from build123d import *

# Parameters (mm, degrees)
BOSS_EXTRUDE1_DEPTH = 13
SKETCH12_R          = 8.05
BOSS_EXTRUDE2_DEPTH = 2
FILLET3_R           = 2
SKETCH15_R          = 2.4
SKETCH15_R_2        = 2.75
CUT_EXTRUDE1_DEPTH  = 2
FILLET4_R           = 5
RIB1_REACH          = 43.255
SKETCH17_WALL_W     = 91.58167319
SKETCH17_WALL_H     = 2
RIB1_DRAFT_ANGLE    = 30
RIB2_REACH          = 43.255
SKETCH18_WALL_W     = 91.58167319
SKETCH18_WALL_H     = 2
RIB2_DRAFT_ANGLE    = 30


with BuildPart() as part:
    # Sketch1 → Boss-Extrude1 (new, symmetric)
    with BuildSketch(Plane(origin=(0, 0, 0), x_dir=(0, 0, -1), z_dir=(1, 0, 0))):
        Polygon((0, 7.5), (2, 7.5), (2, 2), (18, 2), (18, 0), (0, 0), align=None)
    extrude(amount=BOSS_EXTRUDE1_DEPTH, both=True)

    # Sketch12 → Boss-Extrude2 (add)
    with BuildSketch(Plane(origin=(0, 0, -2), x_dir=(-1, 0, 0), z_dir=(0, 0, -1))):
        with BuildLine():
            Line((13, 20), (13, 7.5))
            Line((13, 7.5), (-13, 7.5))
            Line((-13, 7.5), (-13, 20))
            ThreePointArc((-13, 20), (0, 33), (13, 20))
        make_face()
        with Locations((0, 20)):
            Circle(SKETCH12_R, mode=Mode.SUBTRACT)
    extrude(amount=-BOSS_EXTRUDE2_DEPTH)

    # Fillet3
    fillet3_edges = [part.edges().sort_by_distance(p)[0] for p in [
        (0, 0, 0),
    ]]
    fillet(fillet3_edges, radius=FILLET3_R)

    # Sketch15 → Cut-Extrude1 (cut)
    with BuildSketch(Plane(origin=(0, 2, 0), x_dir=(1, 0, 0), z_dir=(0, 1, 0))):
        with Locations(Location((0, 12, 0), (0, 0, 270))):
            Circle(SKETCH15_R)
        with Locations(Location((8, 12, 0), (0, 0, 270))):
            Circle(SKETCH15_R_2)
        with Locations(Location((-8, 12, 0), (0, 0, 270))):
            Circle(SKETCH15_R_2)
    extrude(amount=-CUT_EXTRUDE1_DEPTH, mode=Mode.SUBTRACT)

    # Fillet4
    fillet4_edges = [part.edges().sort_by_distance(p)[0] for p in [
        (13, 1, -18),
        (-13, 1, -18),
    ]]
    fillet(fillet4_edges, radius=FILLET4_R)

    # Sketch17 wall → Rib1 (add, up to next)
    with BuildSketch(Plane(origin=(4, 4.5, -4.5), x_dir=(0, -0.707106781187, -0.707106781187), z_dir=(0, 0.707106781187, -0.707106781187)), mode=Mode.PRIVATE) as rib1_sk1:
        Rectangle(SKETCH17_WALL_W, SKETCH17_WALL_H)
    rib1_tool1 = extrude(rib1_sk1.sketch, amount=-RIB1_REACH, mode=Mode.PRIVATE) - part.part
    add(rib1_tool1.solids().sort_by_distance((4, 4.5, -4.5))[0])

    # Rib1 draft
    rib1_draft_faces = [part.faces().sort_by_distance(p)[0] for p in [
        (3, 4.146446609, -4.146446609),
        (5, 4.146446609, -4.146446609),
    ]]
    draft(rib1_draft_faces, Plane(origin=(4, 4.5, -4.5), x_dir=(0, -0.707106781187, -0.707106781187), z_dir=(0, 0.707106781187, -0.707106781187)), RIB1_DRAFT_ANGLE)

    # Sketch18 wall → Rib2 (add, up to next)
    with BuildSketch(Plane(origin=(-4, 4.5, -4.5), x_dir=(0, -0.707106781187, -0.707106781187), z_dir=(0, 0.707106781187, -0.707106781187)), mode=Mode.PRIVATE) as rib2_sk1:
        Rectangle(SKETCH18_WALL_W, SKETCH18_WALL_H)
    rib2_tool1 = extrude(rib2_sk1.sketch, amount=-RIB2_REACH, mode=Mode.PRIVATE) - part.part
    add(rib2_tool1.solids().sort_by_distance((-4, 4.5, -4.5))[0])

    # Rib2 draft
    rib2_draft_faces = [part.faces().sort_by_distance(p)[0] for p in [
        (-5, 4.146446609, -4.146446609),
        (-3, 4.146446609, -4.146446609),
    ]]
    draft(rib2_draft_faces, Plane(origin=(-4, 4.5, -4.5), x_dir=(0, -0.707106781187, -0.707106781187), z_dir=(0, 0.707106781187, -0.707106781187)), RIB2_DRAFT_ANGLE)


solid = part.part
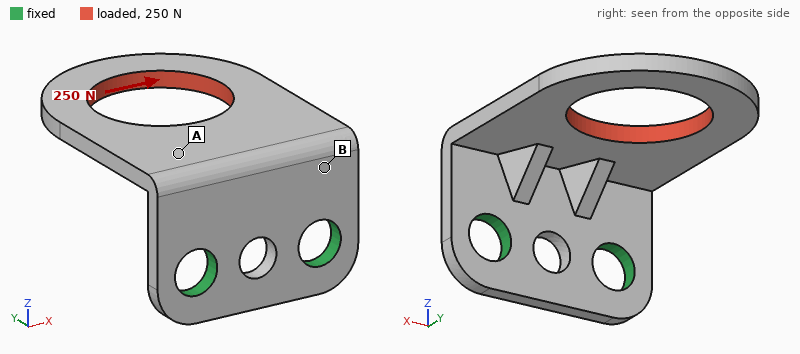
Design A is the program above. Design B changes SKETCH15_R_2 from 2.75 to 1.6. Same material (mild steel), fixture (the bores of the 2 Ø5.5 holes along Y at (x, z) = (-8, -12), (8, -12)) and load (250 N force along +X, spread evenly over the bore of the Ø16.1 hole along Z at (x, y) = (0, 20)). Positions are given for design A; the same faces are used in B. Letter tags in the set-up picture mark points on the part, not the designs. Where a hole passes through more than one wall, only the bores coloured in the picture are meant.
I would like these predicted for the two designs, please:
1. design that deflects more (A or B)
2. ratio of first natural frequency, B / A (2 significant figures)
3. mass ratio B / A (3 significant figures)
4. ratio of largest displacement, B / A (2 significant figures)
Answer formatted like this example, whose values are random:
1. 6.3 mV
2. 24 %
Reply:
1. B
2. 0.93
3. 1.03
4. 1.3
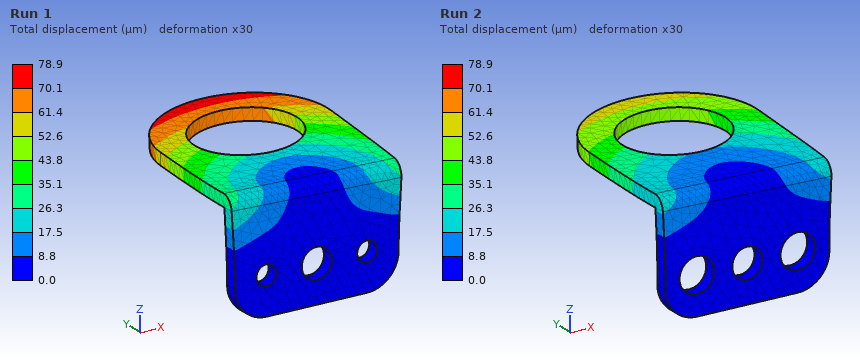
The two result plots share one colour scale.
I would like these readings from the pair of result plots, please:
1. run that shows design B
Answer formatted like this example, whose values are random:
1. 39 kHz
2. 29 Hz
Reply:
1. Run 1
